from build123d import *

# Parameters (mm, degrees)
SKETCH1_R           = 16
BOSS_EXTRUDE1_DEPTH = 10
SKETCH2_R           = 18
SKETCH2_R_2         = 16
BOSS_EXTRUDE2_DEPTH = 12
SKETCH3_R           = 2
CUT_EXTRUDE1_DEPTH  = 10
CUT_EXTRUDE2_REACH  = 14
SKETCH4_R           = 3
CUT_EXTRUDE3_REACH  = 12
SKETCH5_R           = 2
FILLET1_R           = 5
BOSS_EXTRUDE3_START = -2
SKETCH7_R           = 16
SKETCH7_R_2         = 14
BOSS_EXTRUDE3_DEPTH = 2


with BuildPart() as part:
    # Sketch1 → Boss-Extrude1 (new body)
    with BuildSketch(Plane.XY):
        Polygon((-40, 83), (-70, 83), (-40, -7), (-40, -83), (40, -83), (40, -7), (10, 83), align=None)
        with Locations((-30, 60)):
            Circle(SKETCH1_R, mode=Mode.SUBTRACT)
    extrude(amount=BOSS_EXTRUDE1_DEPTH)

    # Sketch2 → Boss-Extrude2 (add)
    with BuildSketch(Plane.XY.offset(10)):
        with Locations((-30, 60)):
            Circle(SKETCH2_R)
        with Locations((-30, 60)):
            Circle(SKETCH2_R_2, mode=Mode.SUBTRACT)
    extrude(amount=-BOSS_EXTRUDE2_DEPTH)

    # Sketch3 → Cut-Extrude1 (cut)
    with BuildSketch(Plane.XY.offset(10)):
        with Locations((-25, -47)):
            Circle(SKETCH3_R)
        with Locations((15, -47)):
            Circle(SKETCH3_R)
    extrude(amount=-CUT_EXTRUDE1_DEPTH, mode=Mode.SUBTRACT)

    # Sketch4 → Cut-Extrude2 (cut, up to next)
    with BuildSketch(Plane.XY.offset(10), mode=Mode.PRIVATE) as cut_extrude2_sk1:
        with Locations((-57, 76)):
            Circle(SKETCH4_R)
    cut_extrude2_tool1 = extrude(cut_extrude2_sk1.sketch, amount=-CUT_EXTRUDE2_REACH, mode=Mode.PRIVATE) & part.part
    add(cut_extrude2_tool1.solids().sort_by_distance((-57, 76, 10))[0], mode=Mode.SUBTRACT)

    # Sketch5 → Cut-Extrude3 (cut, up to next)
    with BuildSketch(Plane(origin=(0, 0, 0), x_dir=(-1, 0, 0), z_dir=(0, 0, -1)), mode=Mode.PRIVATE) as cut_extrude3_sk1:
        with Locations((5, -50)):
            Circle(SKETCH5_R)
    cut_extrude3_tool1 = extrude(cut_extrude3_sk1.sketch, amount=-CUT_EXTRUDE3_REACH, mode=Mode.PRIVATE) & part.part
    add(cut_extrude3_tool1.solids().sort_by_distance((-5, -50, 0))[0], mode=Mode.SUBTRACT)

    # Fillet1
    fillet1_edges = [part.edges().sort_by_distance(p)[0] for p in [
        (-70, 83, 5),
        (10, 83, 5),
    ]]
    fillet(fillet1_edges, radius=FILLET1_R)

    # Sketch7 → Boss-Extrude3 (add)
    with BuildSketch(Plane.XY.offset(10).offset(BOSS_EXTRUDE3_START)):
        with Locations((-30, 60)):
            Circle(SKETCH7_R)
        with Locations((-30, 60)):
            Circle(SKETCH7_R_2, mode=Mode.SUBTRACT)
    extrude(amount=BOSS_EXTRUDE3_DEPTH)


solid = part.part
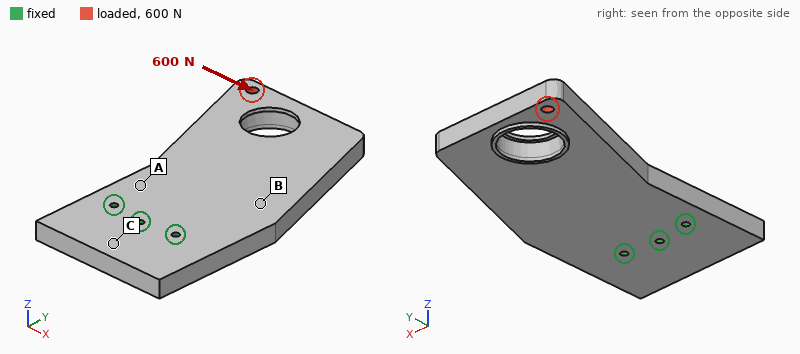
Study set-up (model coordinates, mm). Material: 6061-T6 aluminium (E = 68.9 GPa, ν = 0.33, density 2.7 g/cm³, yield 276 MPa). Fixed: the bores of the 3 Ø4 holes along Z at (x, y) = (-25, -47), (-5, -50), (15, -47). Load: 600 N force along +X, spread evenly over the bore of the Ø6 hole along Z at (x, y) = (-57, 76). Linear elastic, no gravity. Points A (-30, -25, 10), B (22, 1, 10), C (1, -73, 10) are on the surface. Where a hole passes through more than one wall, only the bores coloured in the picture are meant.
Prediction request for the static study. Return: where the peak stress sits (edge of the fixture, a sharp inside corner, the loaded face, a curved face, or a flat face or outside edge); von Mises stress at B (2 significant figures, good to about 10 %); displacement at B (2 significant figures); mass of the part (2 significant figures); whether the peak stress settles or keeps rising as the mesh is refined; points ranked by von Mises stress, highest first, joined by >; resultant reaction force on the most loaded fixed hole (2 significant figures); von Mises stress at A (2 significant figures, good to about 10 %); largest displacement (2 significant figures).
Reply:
edge of the fixture
3.1 MPa
8.9 µm
340 g
keeps rising
A > B > C
1.8 kN
5.0 MPa
38 µm
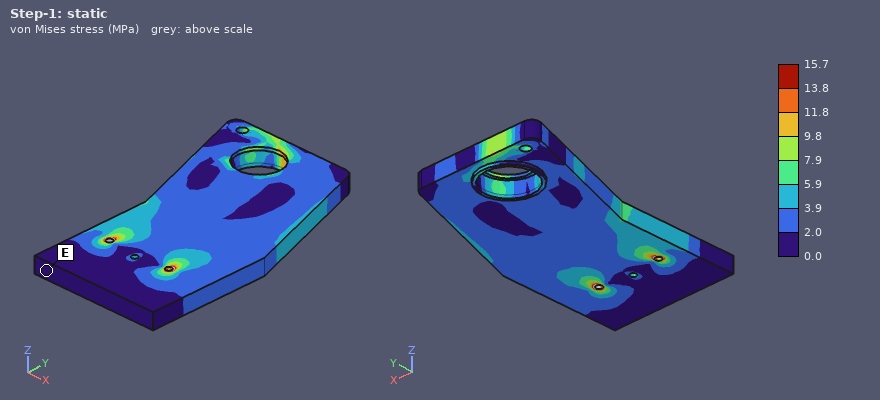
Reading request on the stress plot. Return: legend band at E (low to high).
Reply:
0.0 to 2.0 MPa
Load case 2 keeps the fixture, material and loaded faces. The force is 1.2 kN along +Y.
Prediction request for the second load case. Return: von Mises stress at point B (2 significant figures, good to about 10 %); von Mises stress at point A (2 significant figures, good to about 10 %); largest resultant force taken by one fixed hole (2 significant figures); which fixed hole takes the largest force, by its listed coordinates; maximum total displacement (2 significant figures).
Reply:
2.5 MPa
7.1 MPa
1.9 kN
(-25, -47)
38 µm
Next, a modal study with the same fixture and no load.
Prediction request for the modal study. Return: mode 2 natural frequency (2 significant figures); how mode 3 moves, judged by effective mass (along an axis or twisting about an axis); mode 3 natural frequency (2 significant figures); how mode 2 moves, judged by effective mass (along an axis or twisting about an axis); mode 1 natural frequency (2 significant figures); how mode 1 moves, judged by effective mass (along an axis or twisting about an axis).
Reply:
1500 Hz
along X
2500 Hz
twisting about Y
500 Hz
along Z
